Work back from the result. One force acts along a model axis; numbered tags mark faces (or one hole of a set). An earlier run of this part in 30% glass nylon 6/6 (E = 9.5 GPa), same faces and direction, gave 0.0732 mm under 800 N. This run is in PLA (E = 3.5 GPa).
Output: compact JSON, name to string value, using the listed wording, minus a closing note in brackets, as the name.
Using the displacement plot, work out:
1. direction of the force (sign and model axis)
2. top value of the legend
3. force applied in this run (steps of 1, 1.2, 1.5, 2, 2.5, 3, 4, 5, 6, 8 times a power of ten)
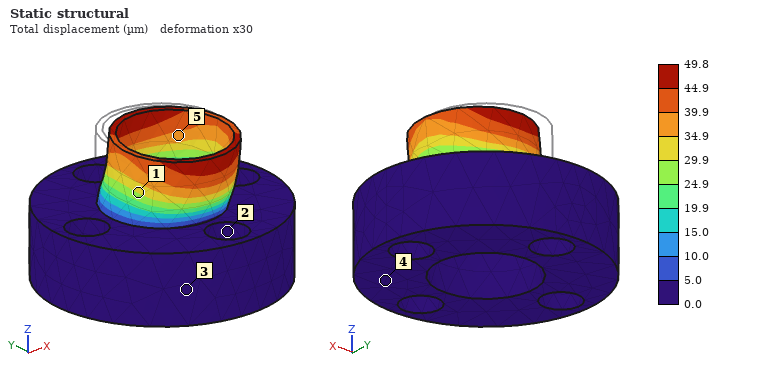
{"direction of the force": "-Y", "top value of the legend": "49.8 µm", "force applied in this run": "200 N"}
